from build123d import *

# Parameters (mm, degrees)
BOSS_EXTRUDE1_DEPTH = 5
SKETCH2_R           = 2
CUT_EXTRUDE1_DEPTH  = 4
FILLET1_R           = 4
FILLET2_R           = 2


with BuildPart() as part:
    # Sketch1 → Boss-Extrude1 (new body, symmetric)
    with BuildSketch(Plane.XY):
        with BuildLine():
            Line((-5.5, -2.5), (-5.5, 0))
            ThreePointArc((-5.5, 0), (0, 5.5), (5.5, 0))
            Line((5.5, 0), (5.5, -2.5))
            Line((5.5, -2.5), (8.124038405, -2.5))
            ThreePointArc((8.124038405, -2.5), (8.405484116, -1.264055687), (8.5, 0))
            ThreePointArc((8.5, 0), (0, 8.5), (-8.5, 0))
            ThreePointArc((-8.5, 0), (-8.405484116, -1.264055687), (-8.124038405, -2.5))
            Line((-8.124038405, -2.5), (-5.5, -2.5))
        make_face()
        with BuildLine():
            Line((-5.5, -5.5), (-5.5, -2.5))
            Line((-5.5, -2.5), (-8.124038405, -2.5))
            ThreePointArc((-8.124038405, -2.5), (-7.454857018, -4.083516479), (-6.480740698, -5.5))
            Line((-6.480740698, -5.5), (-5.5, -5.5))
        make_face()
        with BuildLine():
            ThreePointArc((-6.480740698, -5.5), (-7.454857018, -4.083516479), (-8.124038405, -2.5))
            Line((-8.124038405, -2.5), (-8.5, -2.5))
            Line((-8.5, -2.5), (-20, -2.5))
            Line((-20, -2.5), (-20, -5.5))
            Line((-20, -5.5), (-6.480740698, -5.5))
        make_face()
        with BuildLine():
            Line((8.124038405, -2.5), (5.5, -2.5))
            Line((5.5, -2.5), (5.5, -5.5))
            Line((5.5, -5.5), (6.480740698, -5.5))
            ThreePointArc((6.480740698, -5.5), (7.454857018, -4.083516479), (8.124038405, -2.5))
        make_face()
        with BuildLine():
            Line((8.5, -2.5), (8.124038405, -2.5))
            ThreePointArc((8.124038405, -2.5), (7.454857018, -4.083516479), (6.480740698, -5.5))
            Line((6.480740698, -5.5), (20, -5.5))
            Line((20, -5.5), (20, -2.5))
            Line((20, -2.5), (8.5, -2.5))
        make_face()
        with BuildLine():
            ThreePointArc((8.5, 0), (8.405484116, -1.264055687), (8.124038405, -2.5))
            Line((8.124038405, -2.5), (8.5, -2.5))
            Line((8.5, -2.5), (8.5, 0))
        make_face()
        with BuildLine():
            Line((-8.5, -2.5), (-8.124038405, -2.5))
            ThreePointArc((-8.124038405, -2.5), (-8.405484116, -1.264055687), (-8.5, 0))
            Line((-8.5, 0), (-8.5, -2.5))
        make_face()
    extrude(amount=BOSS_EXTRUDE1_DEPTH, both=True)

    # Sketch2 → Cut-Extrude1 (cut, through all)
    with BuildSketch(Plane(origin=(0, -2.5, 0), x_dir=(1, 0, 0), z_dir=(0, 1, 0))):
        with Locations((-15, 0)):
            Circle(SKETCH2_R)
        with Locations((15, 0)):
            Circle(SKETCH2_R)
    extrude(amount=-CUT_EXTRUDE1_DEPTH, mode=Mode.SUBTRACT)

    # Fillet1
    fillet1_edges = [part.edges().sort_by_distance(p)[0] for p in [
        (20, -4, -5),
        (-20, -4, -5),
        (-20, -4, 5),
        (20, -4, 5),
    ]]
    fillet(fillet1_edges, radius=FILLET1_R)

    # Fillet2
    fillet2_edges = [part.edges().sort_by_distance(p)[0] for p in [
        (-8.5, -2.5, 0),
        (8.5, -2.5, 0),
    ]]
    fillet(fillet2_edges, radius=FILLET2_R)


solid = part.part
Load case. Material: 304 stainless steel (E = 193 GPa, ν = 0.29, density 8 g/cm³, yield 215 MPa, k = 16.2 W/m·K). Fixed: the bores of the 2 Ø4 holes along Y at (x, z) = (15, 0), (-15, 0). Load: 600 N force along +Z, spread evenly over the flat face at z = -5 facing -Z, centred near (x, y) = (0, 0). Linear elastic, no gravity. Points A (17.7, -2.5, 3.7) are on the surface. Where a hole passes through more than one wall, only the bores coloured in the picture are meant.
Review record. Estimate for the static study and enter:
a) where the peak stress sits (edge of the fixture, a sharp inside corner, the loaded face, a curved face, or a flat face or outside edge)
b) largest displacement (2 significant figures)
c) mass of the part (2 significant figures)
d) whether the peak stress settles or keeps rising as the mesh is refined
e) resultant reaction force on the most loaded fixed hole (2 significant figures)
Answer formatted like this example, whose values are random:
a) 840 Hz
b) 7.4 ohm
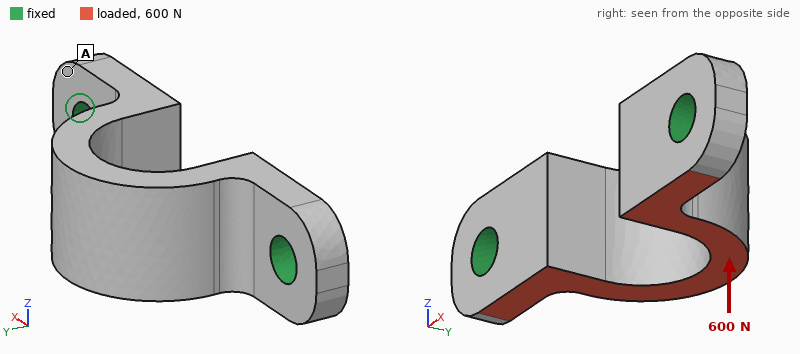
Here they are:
a) edge of the fixture
b) 16 µm
c) 13 g
d) keeps rising
e) 300 N
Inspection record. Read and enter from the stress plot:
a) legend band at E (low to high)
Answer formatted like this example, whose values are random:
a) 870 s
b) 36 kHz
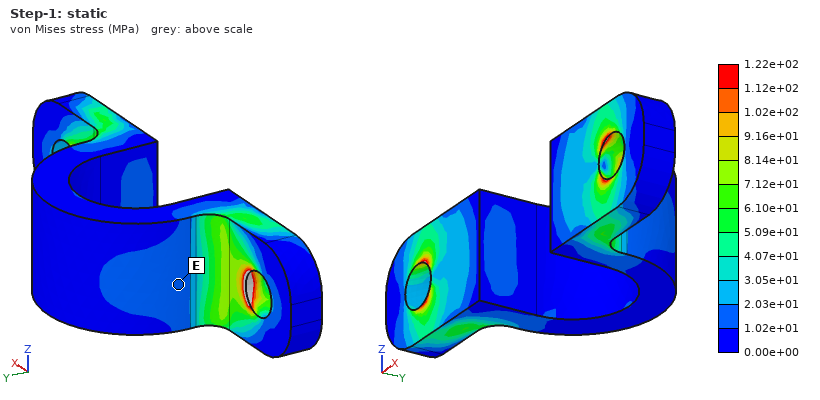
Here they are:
a) 1.02e+01 to 2.03e+01 MPa
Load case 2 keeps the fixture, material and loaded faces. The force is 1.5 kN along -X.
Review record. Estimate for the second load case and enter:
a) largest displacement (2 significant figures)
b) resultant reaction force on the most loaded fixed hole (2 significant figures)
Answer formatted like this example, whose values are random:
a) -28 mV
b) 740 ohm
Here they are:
a) 14 µm
b) 800 N
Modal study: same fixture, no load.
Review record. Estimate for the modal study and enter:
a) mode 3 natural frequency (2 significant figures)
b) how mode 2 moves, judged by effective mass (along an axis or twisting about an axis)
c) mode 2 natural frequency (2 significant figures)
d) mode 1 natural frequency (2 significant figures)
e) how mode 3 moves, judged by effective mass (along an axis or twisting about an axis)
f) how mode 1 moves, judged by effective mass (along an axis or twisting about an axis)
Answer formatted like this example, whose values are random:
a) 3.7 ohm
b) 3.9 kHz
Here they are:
a) 23 kHz
b) along X
c) 21 kHz
d) 11 kHz
e) along Y
f) along Z
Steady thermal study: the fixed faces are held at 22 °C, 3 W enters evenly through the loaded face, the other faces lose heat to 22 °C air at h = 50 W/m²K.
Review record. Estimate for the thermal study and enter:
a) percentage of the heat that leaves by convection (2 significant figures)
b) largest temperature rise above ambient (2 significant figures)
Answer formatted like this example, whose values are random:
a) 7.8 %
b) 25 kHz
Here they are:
a) 22 %
b) 24 K
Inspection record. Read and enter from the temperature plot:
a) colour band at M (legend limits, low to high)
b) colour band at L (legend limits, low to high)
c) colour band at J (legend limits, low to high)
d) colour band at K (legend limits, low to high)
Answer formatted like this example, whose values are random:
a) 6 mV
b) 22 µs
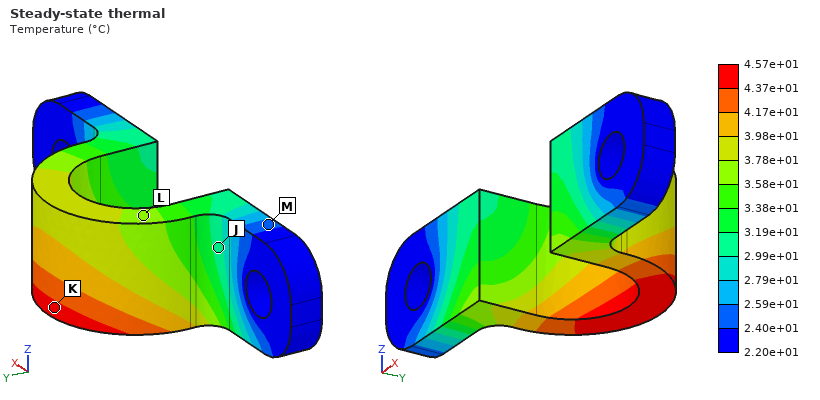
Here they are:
a) 2.40e+01 to 2.59e+01 °C
b) 3.58e+01 to 3.78e+01 °C
c) 2.99e+01 to 3.19e+01 °C
d) 4.37e+01 to 4.57e+01 °C
